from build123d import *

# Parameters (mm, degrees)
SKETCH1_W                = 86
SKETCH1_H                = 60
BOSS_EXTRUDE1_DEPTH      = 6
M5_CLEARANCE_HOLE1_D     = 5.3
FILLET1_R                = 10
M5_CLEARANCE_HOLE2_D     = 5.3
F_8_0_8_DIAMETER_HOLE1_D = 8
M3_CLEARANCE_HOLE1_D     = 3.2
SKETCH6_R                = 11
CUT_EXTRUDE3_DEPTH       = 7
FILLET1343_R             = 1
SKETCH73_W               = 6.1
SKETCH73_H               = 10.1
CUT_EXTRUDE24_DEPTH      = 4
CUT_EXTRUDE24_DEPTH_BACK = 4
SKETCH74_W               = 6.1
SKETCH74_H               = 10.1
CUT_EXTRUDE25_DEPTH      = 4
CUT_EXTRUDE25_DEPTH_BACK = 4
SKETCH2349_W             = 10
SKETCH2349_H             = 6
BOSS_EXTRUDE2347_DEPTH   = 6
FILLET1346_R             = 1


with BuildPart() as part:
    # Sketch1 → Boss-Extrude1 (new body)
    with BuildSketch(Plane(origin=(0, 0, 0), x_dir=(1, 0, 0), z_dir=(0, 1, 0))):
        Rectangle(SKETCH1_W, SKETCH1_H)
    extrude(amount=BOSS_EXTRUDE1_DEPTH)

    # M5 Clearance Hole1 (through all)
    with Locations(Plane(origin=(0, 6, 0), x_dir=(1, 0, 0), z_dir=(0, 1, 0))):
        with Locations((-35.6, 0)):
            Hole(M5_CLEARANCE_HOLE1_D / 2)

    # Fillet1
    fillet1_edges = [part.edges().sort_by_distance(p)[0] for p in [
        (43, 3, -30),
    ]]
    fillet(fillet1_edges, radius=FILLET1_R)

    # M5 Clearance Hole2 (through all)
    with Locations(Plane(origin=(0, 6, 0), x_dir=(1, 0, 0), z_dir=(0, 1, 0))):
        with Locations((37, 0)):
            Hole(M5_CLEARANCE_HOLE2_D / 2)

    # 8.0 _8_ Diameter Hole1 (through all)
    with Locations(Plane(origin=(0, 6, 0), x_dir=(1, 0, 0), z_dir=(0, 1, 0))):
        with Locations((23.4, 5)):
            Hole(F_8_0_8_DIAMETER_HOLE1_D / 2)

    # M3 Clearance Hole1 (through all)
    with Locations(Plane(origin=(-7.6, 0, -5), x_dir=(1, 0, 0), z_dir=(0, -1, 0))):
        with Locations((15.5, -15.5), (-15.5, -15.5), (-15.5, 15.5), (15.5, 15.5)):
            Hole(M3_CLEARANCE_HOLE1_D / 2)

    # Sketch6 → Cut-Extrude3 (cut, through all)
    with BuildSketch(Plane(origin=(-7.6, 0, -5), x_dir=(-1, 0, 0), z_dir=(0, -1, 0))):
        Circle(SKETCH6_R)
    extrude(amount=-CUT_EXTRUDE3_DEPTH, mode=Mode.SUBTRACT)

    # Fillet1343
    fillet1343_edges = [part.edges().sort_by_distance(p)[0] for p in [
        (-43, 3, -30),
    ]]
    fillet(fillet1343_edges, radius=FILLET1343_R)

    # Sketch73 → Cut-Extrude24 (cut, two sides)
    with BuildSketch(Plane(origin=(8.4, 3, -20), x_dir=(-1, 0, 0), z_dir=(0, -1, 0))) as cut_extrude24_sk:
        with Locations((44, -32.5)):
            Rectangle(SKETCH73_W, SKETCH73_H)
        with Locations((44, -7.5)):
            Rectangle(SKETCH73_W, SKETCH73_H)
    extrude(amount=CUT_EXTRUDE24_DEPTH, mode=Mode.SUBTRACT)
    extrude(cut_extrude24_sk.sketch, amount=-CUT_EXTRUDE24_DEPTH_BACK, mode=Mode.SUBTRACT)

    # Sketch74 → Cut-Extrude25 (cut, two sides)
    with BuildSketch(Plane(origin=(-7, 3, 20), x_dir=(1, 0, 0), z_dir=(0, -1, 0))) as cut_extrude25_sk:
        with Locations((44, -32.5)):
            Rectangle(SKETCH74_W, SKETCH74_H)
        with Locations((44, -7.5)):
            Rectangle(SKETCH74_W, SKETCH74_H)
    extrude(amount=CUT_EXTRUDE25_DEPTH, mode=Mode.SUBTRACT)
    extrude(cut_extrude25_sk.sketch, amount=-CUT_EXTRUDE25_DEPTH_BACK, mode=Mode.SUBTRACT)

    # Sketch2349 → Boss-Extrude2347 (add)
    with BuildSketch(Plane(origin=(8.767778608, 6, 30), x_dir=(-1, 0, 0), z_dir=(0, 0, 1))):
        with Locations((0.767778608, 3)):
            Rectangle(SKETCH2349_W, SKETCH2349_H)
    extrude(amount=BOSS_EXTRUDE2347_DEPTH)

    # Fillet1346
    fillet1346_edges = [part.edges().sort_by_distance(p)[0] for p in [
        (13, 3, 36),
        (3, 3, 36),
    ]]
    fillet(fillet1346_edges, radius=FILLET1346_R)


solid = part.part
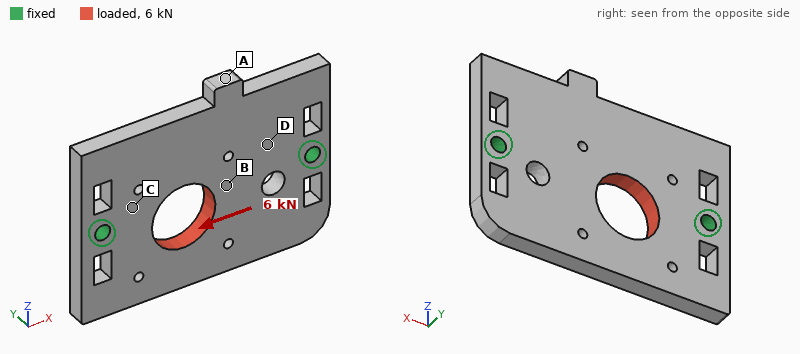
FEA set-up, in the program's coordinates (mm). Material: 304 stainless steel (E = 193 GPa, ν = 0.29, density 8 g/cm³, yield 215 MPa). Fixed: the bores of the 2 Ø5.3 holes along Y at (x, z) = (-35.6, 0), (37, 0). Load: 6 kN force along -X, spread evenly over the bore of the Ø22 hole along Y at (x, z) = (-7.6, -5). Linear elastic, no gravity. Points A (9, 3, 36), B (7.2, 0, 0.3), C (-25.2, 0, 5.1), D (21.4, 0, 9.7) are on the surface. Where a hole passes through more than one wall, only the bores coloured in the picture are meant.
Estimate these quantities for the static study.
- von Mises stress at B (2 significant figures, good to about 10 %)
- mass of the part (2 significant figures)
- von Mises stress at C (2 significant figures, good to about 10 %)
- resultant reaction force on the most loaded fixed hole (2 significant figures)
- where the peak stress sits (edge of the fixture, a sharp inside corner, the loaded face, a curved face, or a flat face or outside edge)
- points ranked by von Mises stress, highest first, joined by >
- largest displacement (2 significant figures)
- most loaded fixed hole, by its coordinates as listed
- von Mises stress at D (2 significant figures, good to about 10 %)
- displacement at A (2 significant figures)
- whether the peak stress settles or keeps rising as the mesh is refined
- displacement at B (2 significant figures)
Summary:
17 MPa
210 g
28 MPa
3.3 kN
edge of the fixture
C > B > D > A
6.3 µm
(-35.6, 0)
9.6 MPa
1.9 µm
keeps rising
3.9 µm
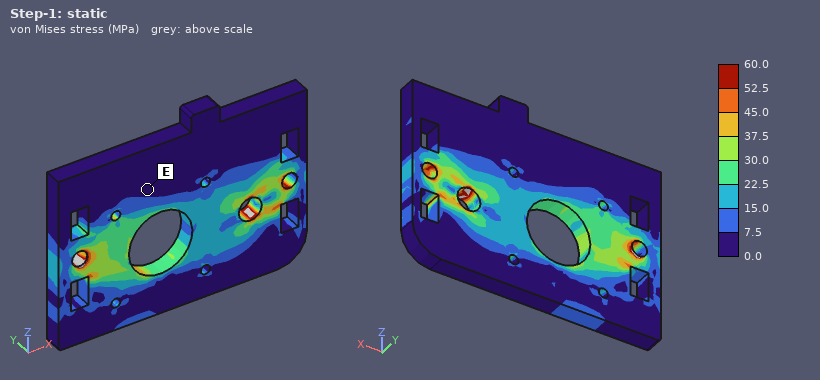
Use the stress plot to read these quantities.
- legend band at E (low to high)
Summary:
0.0 to 7.5 MPa
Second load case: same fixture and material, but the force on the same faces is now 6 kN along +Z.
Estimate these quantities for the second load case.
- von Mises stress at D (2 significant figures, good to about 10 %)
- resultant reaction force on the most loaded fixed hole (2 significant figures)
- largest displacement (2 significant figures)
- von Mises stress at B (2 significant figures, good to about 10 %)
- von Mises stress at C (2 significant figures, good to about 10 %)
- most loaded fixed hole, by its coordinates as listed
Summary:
18 MPa
3.7 kN
8.5 µm
15 MPa
27 MPa
(-35.6, 0)
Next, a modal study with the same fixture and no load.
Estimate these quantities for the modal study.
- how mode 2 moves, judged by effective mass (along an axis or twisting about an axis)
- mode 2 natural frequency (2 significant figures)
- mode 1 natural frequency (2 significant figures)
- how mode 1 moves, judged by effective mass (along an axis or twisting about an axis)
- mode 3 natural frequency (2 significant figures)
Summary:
along Y
3300 Hz
2600 Hz
twisting about X
5500 Hz
